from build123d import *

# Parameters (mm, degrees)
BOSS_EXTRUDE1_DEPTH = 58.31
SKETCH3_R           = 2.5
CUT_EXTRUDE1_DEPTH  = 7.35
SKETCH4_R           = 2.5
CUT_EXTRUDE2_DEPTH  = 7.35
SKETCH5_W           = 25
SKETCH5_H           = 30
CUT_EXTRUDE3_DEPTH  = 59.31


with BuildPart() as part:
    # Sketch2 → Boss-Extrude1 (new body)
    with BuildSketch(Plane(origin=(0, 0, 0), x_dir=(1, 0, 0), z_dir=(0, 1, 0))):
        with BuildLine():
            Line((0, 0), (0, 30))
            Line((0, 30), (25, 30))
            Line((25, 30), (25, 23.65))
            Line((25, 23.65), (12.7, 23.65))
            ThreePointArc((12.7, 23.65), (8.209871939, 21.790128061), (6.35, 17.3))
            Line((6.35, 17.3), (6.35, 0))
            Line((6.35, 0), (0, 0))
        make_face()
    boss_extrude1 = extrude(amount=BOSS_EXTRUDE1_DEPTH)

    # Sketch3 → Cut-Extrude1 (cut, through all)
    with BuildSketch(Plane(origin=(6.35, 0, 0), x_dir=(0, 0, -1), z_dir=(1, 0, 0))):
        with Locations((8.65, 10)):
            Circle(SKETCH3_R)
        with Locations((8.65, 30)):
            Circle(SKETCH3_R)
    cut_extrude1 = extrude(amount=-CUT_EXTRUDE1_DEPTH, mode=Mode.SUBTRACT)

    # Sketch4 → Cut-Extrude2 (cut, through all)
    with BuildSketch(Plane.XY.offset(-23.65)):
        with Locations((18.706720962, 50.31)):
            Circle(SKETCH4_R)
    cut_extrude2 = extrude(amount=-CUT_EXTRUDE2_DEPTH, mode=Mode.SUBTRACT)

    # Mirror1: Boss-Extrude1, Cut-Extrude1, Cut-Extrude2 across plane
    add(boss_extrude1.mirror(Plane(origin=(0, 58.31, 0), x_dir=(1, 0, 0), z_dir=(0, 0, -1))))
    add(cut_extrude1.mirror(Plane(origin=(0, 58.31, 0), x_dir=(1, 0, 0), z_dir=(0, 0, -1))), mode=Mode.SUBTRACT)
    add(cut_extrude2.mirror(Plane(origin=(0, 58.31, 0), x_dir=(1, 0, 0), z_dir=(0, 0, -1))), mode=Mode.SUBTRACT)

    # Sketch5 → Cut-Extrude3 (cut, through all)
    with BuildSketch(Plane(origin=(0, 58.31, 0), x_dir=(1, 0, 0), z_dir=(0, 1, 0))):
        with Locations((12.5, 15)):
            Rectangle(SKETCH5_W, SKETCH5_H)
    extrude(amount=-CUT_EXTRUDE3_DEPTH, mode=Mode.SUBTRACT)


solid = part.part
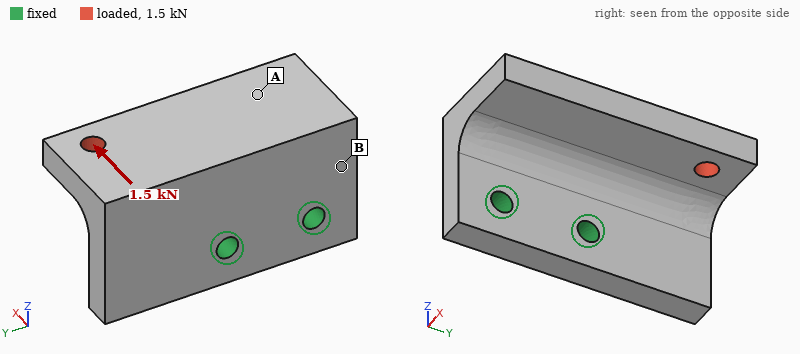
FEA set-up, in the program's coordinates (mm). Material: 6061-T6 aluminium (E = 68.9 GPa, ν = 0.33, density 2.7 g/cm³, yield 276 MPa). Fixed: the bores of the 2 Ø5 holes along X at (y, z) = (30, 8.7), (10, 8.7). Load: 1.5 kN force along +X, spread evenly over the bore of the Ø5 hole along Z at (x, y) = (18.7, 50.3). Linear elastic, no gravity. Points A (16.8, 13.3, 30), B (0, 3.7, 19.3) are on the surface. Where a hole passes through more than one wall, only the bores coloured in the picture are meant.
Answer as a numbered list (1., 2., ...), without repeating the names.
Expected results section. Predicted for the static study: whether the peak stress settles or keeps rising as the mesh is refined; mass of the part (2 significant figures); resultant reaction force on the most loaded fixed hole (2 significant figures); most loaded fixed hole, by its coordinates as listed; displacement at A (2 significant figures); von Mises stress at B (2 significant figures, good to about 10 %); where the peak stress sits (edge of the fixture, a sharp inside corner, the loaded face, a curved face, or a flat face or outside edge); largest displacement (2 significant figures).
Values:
1. keeps rising
2. 49 g
3. 2.3 kN
4. (30, 8.7)
5. 0.059 mm
6. 50 MPa
7. edge of the fixture
8. 0.23 mm
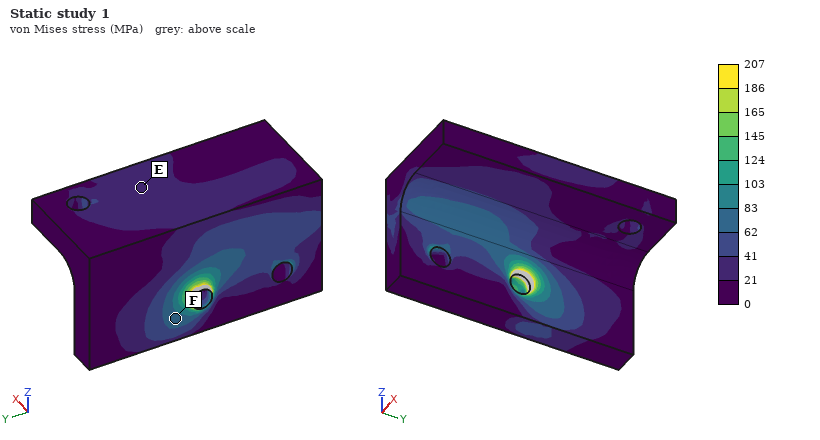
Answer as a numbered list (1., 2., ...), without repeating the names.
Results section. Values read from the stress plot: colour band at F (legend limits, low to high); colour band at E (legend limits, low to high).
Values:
1. 62 to 83 MPa
2. 21 to 41 MPa
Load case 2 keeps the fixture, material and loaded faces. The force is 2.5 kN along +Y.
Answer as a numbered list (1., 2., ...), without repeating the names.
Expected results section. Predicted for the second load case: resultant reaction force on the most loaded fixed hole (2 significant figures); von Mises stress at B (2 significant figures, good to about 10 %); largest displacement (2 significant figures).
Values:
1. 2.6 kN
2. 22 MPa
3. 0.13 mm
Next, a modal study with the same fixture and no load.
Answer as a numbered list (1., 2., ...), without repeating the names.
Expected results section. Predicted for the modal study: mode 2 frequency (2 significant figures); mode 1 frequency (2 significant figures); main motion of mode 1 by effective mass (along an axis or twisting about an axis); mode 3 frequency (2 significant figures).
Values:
1. 5500 Hz
2. 3800 Hz
3. along X
4. 8800 Hz
